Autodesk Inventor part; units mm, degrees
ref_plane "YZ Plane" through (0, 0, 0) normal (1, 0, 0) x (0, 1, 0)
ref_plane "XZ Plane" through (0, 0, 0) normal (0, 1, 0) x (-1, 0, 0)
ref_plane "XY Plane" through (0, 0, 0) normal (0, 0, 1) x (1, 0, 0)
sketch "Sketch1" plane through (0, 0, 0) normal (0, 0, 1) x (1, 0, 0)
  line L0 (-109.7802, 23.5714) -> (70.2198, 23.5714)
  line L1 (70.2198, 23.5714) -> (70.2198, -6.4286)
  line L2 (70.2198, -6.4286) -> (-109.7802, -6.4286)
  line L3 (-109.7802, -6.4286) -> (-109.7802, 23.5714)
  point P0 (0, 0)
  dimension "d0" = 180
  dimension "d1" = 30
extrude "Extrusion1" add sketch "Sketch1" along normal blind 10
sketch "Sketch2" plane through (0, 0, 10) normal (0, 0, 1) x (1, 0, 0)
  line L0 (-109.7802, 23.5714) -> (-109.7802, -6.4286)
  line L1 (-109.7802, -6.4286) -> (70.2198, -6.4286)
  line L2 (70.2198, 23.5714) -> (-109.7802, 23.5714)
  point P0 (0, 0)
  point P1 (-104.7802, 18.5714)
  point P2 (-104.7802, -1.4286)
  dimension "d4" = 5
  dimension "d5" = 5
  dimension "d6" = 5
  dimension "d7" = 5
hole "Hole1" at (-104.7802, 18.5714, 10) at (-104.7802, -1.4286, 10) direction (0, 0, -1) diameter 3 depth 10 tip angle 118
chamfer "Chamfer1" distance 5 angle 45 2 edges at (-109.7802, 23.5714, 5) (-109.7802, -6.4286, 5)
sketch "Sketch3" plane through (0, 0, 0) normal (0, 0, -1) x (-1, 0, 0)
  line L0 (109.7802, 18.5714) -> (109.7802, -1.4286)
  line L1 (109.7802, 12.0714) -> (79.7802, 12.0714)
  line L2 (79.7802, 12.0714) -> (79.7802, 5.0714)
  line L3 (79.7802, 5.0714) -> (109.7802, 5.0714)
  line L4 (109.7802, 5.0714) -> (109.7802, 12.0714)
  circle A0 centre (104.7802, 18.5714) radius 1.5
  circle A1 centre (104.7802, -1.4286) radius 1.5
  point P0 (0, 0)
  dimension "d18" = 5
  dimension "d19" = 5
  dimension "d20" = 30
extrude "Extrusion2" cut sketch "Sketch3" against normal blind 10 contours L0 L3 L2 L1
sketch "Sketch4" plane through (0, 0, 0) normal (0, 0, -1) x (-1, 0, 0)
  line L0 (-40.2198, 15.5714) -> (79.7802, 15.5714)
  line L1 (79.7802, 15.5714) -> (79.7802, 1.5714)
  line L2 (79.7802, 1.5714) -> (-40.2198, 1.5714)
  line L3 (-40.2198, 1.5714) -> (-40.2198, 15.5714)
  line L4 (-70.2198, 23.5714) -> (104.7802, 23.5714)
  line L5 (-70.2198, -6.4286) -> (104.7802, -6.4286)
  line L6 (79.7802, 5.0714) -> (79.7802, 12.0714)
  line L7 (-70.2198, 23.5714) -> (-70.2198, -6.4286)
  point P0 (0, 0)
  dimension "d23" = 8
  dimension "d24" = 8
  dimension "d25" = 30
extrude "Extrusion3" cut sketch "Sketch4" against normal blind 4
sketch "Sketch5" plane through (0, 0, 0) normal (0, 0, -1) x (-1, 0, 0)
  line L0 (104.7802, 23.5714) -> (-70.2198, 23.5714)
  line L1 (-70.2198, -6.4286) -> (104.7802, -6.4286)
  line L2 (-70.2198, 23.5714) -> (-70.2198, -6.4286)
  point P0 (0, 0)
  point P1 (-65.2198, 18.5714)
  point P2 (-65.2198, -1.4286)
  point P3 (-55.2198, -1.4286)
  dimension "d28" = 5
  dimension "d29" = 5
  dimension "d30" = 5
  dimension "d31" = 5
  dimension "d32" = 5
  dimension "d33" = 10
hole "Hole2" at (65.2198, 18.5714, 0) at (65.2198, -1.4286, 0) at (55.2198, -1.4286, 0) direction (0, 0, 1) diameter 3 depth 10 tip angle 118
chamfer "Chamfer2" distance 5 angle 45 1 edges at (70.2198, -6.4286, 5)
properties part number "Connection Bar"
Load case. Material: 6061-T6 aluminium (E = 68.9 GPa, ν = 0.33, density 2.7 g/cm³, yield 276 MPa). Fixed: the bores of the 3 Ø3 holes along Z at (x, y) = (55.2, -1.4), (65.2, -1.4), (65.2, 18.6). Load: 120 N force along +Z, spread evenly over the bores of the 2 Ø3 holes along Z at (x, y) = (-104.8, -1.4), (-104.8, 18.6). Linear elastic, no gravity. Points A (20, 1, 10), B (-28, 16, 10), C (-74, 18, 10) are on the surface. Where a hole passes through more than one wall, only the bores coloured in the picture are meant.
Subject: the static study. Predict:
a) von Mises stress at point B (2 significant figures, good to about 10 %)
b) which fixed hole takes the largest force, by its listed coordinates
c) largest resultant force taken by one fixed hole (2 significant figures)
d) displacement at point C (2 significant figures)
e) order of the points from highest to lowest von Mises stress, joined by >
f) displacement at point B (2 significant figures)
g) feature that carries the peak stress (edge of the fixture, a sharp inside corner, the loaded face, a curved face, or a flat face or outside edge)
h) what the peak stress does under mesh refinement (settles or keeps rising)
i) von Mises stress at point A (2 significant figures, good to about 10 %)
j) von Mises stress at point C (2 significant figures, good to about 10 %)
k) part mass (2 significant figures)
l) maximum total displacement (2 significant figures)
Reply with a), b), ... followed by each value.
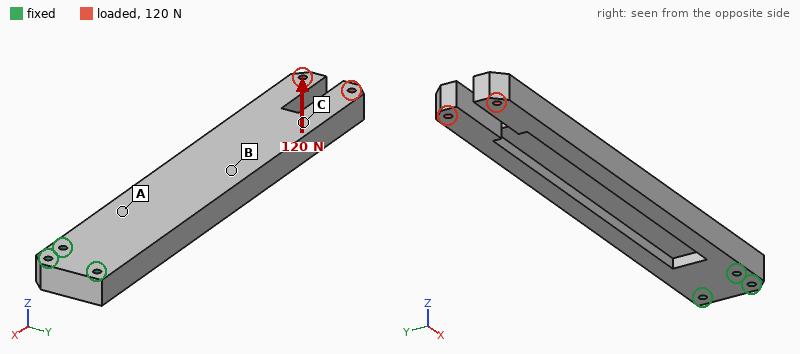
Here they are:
a) 22 MPa
b) (55.2, -1.4)
c) 610 N
d) 0.95 mm
e) A > B > C
f) 0.45 mm
g) edge of the fixture
h) keeps rising
i) 36 MPa
j) 11 MPa
k) 120 g
l) 1.4 mm
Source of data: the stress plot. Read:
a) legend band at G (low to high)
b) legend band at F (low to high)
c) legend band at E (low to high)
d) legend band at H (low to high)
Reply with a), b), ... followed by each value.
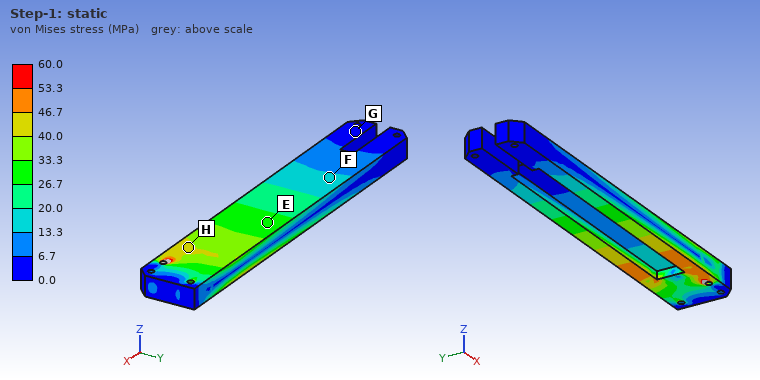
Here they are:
a) 0.0 to 6.7 MPa
b) 13.3 to 20.0 MPa
c) 26.7 to 33.3 MPa
d) 40.0 to 46.7 MPa
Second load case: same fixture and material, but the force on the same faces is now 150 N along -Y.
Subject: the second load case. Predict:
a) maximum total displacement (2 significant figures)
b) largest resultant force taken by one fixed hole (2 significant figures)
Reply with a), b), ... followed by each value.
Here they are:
a) 0.18 mm
b) 1.0 kN
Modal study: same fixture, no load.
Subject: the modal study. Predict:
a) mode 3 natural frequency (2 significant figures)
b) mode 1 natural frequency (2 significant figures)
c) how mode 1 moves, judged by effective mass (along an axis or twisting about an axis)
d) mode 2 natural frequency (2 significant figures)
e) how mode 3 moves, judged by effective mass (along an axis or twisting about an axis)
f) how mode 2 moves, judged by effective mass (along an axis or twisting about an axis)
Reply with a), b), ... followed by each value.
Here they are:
a) 1700 Hz
b) 290 Hz
c) along Z
d) 910 Hz
e) along Z
f) along Y
